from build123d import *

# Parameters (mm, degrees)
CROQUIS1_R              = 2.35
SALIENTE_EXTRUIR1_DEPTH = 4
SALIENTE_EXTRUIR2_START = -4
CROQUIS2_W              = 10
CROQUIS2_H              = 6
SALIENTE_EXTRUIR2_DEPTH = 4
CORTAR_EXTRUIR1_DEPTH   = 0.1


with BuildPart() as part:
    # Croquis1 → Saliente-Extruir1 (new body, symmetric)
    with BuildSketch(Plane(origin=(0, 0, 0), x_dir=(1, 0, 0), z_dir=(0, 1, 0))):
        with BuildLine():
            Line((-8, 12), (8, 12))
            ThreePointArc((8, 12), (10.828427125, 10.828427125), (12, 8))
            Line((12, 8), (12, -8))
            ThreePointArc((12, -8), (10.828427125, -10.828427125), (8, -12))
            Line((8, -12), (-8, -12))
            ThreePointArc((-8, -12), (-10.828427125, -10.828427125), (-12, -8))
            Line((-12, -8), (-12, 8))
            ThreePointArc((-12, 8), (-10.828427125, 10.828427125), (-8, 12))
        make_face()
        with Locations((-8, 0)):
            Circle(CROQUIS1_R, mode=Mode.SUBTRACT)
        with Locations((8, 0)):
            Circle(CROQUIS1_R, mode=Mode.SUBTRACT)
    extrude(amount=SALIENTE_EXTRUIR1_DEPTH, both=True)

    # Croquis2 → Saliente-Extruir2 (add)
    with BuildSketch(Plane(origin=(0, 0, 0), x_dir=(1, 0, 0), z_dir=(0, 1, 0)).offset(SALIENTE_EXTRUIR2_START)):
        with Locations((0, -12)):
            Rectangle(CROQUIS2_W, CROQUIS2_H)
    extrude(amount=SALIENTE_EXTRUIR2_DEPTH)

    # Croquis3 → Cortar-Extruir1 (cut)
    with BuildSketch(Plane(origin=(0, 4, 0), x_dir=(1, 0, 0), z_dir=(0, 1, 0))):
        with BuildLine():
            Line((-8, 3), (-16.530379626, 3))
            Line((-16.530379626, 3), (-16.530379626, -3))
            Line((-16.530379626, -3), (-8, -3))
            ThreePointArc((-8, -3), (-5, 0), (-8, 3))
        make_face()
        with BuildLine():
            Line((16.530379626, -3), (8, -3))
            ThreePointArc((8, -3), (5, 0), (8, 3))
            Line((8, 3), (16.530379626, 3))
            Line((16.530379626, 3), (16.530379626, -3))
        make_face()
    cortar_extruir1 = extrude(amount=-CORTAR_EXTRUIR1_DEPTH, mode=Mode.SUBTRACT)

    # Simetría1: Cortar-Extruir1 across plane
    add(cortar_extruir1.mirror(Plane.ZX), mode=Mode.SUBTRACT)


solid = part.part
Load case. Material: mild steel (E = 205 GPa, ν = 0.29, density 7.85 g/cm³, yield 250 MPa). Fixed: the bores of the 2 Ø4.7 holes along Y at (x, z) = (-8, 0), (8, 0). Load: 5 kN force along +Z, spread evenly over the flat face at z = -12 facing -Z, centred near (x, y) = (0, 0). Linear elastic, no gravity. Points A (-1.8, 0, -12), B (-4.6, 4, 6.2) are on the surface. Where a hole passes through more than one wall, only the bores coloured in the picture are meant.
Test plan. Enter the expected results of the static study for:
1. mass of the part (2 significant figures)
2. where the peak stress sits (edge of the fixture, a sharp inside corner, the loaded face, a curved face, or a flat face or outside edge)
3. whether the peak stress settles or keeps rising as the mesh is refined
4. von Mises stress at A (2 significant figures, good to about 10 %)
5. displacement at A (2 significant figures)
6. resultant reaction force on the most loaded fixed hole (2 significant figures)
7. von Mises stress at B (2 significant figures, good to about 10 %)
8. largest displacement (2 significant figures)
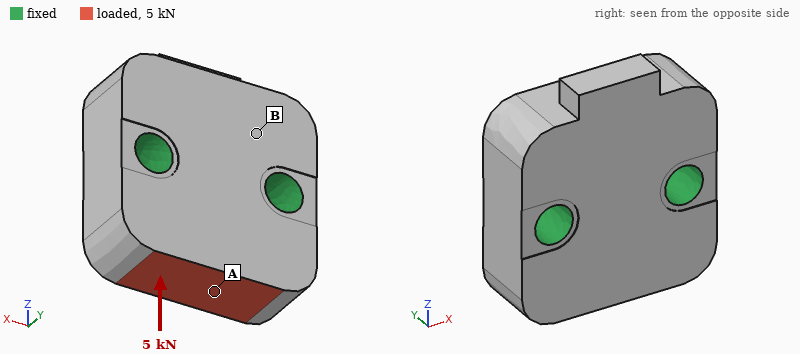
34 g
edge of the fixture
keeps rising
34 MPa
2.2 µm
2.6 kN
7.5 MPa
2.3 µm
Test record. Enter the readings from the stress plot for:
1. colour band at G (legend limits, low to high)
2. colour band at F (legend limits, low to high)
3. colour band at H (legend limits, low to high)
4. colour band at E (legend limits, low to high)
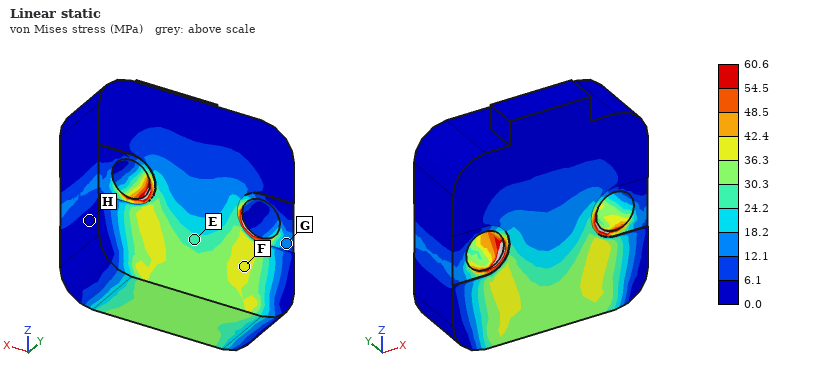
12.1 to 18.2 MPa
36.3 to 42.4 MPa
0.0 to 6.1 MPa
24.2 to 30.3 MPa
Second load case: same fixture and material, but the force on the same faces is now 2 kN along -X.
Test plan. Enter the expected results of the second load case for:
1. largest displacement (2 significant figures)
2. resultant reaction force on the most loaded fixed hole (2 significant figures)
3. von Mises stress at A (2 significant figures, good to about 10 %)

2.2 µm
1.6 kN
27 MPa
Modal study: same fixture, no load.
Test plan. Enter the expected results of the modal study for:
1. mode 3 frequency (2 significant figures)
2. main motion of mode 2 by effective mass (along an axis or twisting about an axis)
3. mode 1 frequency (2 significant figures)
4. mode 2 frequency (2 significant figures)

57 kHz
along Y
34 kHz
41 kHz
